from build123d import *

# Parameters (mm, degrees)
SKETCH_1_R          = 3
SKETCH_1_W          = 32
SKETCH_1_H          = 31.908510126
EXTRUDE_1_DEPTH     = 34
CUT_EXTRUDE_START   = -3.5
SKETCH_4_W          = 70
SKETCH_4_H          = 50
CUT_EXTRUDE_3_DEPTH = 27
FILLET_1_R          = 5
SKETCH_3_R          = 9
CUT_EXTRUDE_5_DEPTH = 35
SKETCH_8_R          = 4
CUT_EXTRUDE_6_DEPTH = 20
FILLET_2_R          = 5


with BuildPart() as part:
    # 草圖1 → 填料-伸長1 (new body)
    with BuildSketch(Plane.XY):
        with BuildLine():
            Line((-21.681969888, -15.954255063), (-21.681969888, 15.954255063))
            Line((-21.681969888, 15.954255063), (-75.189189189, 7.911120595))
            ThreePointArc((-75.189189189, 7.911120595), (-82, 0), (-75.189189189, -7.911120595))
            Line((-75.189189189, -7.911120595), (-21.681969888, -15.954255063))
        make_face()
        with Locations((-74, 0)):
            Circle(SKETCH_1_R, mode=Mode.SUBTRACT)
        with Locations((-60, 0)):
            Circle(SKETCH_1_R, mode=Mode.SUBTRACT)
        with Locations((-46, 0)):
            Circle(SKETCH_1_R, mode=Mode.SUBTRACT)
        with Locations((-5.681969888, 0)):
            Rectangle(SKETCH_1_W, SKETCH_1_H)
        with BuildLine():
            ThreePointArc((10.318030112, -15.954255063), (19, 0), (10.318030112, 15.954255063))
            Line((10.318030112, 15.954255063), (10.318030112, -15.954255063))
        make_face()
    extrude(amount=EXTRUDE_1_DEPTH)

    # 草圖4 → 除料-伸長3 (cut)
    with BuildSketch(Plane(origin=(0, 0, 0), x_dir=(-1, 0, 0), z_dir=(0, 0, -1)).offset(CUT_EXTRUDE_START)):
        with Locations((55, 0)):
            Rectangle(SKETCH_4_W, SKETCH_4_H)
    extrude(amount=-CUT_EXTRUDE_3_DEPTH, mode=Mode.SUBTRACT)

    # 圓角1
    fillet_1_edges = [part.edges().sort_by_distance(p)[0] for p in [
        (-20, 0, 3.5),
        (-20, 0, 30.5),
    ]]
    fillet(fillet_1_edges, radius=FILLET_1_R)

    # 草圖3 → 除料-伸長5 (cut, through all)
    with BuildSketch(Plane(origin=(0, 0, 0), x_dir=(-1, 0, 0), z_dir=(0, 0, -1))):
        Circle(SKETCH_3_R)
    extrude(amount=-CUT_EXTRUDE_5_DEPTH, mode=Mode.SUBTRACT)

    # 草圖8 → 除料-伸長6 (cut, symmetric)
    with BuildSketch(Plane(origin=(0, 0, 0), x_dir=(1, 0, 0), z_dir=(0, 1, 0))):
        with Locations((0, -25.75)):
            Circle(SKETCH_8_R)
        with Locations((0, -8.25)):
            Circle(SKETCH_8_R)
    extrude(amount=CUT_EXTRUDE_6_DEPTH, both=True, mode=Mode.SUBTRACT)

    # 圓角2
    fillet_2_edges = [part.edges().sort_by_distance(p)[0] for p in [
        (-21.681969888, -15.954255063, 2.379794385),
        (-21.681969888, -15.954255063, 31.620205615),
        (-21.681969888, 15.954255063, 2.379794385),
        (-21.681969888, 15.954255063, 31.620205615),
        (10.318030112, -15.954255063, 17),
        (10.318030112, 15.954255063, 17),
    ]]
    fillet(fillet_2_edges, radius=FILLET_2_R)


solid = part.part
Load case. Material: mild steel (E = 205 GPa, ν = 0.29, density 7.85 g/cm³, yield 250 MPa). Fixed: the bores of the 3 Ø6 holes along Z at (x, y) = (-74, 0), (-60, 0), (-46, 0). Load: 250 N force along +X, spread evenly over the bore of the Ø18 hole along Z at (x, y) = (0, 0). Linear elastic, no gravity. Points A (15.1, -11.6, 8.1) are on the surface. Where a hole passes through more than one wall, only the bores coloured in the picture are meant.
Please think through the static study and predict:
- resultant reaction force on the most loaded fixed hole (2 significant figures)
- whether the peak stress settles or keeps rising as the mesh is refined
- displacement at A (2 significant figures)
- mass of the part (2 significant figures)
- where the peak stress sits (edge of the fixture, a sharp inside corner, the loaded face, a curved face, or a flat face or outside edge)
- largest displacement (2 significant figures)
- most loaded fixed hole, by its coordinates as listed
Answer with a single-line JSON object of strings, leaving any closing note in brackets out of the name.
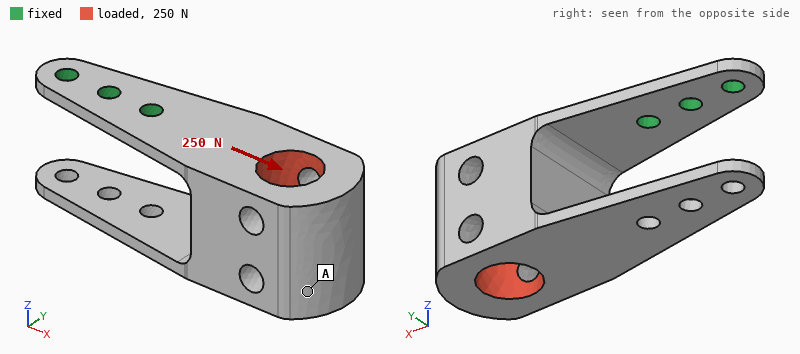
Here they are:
{"resultant reaction force on the most loaded fixed hole": "210 N", "whether the peak stress settles or keeps rising as the mesh is refined": "keeps rising", "displacement at A": "0.23 mm", "mass of the part": "310 g", "where the peak stress sits": "edge of the fixture", "largest displacement": "0.26 mm", "most loaded fixed hole, by its coordinates as listed": "(-46, 0)"}
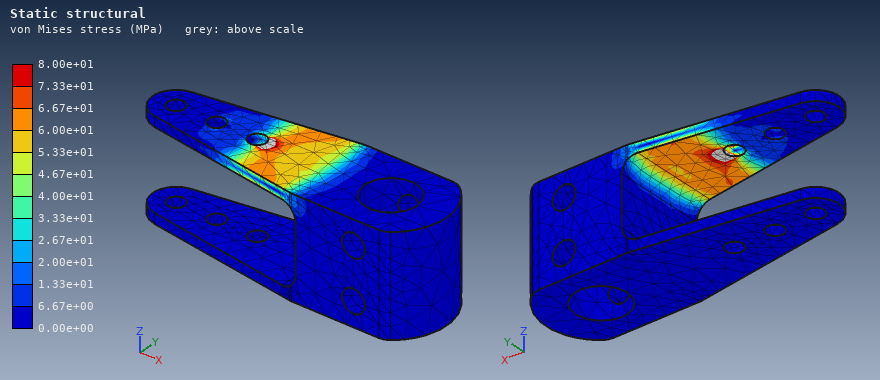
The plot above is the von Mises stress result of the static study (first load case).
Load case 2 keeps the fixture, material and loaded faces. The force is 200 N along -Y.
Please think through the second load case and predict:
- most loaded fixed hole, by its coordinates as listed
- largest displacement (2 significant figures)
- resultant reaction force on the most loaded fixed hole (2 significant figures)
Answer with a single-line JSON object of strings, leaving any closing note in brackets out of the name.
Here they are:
{"most loaded fixed hole, by its coordinates as listed": "(-46, 0)", "largest displacement": "74 µm", "resultant reaction force on the most loaded fixed hole": "530 N"}
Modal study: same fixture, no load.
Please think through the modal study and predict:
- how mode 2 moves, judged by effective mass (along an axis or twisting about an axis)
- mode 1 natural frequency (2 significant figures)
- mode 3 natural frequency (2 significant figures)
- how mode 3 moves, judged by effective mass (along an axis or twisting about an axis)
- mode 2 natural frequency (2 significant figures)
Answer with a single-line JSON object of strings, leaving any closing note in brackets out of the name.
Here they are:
{"how mode 2 moves, judged by effective mass": "along Y", "mode 1 natural frequency": "240 Hz", "mode 3 natural frequency": "1000 Hz", "how mode 3 moves, judged by effective mass": "along Z", "mode 2 natural frequency": "550 Hz"}
